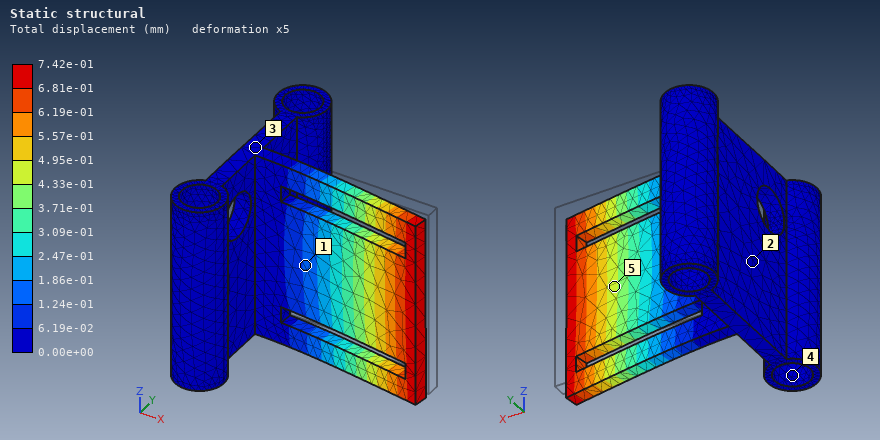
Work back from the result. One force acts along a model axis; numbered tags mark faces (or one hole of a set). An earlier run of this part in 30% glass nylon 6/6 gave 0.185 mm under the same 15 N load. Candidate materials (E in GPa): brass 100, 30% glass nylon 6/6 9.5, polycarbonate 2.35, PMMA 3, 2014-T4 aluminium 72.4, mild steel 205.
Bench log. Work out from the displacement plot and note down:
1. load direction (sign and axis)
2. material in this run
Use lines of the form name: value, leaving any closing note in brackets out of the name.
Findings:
load direction: -Y
material in this run: polycarbonate
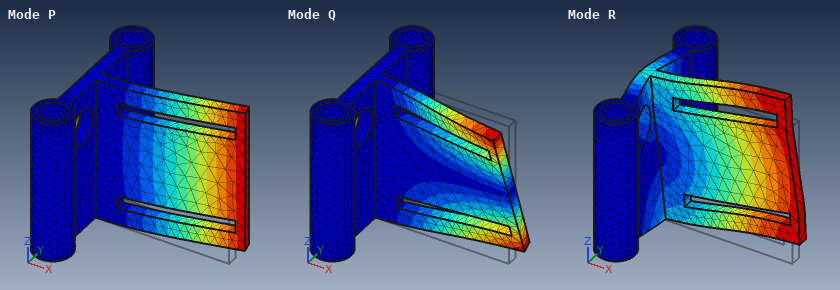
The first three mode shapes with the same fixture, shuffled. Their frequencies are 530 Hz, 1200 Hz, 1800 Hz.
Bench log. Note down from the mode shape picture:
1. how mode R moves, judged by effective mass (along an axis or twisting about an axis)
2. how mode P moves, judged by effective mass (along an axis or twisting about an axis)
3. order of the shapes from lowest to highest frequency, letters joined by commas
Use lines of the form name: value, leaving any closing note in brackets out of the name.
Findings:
how mode R moves, judged by effective mass: along Z
how mode P moves, judged by effective mass: along Y
order of the shapes from lowest to highest frequency, letters joined by commas: P, Q, R
